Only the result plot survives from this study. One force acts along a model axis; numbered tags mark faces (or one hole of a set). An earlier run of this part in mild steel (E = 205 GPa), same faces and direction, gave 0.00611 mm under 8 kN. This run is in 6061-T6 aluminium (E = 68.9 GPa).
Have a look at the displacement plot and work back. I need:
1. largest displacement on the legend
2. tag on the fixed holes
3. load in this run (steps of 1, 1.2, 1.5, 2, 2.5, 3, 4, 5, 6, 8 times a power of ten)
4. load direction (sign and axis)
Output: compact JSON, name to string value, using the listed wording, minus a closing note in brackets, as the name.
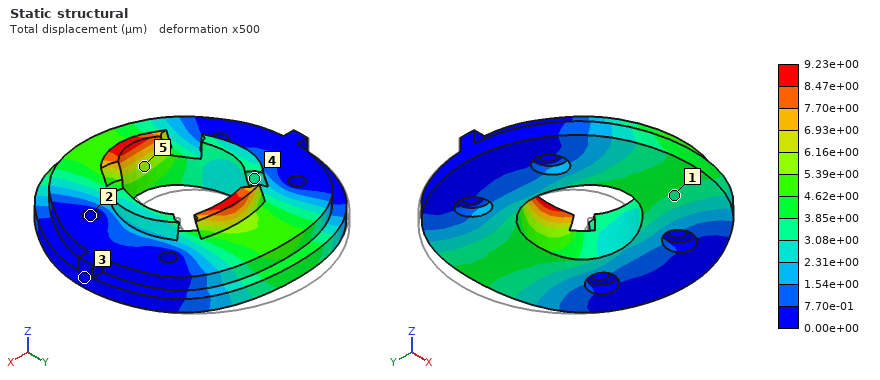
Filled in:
{"largest displacement on the legend": "9.23e+00 µm", "tag on the fixed holes": "2", "load in this run": "4 kN", "load direction": "-Y"}
